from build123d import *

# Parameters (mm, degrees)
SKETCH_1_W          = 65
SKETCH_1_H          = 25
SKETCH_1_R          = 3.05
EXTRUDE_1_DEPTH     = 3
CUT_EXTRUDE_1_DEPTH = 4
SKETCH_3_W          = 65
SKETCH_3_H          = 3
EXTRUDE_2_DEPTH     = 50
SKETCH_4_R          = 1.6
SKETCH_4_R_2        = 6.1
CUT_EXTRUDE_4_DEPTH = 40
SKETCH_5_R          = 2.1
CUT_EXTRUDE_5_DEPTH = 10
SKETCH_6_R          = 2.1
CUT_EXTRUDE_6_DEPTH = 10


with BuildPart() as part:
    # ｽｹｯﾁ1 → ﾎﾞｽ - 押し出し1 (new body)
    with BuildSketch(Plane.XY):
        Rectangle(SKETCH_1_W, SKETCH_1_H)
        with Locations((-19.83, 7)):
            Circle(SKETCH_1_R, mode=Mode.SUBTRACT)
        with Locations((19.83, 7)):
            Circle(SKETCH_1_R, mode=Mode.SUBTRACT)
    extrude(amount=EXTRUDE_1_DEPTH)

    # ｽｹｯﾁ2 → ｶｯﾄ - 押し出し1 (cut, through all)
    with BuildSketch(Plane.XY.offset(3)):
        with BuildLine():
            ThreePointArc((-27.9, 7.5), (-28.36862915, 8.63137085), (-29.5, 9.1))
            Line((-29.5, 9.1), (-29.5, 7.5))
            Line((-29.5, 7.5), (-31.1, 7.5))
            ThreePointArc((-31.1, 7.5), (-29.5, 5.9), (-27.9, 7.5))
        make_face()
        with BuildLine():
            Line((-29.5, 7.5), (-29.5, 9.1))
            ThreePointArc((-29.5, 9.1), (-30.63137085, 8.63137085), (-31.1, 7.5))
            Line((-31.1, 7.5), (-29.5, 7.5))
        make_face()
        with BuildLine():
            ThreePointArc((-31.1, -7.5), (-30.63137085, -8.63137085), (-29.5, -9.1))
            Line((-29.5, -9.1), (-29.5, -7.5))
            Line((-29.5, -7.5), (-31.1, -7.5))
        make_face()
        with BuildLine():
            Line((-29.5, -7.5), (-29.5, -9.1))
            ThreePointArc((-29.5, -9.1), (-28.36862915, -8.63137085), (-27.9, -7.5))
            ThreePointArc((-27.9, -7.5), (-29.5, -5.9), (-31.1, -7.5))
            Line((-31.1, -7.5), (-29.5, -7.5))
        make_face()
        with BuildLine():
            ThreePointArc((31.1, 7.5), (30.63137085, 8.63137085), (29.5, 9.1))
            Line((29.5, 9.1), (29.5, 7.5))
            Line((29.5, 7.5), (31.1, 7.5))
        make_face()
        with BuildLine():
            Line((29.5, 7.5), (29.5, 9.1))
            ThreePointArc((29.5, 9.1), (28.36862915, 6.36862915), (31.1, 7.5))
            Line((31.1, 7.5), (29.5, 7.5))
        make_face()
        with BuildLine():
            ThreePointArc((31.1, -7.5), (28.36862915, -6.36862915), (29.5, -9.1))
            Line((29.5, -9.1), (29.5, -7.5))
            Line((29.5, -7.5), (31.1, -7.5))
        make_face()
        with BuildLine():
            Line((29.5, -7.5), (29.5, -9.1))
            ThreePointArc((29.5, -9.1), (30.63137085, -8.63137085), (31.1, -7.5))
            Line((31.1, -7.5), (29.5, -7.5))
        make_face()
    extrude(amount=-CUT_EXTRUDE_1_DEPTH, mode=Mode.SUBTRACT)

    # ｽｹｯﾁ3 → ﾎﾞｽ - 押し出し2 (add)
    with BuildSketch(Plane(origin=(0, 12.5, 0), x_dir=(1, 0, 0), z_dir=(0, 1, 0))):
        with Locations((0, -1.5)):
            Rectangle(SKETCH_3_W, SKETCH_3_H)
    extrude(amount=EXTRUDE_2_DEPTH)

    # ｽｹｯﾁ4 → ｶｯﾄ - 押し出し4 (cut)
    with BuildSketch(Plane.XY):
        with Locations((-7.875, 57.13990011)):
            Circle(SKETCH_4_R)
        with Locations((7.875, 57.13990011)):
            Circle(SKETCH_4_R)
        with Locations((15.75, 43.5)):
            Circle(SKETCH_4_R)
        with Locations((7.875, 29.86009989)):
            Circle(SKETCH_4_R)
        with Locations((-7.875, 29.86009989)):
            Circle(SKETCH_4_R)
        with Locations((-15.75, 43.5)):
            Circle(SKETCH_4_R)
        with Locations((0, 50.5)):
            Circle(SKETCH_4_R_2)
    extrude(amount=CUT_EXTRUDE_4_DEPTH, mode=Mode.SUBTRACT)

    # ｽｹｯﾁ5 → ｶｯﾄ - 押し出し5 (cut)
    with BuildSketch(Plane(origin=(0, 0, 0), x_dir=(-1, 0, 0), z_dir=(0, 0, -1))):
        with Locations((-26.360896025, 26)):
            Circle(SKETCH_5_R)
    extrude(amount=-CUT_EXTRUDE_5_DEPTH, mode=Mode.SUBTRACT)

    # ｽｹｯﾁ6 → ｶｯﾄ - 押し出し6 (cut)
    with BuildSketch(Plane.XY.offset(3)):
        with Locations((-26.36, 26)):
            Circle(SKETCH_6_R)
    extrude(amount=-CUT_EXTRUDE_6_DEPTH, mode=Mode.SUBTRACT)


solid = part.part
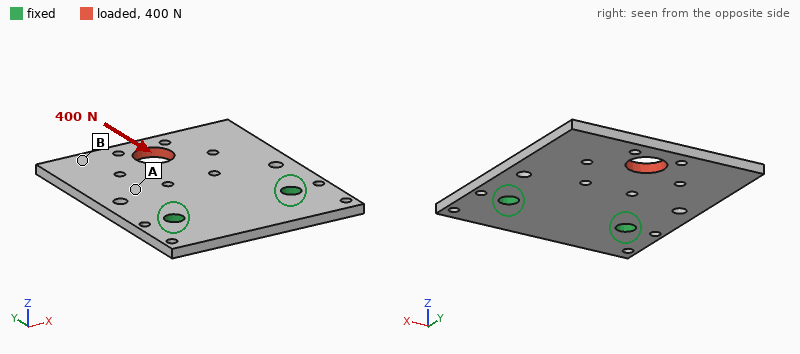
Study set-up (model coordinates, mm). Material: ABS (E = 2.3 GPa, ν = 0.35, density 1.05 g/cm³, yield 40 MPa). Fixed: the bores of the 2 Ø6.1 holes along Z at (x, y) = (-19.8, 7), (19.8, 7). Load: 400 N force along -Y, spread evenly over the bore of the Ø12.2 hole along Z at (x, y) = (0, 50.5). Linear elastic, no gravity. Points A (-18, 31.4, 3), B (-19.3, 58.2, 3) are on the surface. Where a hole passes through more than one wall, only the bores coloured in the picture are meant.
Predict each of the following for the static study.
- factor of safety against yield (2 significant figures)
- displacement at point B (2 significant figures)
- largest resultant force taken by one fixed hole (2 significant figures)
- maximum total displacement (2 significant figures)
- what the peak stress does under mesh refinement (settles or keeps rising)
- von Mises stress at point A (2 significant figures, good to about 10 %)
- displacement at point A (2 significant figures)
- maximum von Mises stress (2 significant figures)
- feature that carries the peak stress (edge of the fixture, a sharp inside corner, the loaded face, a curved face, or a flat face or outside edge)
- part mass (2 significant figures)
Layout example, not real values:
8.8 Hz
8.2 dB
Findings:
3.2
0.042 mm
200 N
0.11 mm
settles
2.6 MPa
0.031 mm
13 MPa
a curved face
14 g
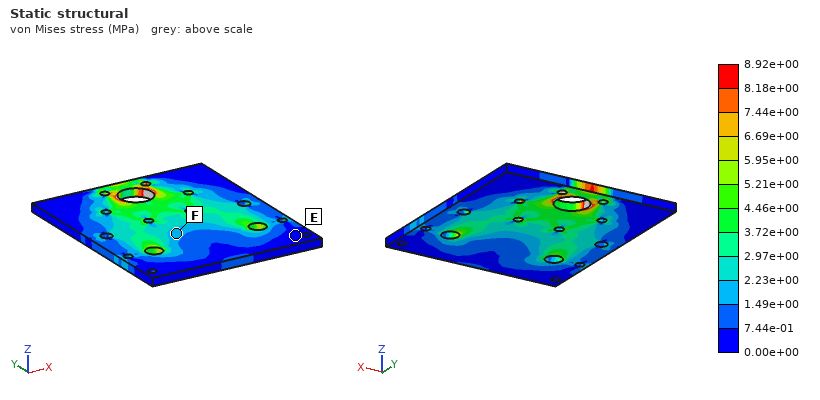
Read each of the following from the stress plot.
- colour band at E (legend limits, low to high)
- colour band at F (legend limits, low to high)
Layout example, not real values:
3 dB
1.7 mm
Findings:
0.00e+00 to 7.44e-01 MPa
1.49e+00 to 2.23e+00 MPa
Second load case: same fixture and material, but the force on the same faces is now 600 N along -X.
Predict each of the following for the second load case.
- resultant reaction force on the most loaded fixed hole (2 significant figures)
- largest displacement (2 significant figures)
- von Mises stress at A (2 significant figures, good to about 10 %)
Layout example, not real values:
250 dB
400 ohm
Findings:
670 N
0.49 mm
6.7 MPa
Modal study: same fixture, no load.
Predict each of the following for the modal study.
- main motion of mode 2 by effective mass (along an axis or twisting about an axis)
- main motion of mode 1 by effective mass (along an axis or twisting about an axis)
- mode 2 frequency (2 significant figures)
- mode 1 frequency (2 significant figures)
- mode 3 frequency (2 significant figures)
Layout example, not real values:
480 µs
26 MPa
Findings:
twisting about Y
along Z
490 Hz
250 Hz
1300 Hz
